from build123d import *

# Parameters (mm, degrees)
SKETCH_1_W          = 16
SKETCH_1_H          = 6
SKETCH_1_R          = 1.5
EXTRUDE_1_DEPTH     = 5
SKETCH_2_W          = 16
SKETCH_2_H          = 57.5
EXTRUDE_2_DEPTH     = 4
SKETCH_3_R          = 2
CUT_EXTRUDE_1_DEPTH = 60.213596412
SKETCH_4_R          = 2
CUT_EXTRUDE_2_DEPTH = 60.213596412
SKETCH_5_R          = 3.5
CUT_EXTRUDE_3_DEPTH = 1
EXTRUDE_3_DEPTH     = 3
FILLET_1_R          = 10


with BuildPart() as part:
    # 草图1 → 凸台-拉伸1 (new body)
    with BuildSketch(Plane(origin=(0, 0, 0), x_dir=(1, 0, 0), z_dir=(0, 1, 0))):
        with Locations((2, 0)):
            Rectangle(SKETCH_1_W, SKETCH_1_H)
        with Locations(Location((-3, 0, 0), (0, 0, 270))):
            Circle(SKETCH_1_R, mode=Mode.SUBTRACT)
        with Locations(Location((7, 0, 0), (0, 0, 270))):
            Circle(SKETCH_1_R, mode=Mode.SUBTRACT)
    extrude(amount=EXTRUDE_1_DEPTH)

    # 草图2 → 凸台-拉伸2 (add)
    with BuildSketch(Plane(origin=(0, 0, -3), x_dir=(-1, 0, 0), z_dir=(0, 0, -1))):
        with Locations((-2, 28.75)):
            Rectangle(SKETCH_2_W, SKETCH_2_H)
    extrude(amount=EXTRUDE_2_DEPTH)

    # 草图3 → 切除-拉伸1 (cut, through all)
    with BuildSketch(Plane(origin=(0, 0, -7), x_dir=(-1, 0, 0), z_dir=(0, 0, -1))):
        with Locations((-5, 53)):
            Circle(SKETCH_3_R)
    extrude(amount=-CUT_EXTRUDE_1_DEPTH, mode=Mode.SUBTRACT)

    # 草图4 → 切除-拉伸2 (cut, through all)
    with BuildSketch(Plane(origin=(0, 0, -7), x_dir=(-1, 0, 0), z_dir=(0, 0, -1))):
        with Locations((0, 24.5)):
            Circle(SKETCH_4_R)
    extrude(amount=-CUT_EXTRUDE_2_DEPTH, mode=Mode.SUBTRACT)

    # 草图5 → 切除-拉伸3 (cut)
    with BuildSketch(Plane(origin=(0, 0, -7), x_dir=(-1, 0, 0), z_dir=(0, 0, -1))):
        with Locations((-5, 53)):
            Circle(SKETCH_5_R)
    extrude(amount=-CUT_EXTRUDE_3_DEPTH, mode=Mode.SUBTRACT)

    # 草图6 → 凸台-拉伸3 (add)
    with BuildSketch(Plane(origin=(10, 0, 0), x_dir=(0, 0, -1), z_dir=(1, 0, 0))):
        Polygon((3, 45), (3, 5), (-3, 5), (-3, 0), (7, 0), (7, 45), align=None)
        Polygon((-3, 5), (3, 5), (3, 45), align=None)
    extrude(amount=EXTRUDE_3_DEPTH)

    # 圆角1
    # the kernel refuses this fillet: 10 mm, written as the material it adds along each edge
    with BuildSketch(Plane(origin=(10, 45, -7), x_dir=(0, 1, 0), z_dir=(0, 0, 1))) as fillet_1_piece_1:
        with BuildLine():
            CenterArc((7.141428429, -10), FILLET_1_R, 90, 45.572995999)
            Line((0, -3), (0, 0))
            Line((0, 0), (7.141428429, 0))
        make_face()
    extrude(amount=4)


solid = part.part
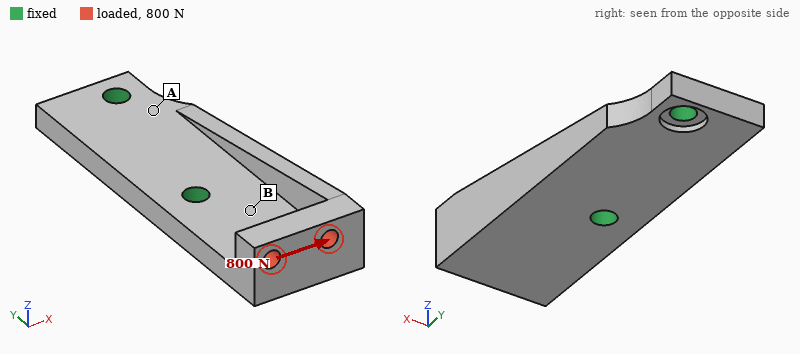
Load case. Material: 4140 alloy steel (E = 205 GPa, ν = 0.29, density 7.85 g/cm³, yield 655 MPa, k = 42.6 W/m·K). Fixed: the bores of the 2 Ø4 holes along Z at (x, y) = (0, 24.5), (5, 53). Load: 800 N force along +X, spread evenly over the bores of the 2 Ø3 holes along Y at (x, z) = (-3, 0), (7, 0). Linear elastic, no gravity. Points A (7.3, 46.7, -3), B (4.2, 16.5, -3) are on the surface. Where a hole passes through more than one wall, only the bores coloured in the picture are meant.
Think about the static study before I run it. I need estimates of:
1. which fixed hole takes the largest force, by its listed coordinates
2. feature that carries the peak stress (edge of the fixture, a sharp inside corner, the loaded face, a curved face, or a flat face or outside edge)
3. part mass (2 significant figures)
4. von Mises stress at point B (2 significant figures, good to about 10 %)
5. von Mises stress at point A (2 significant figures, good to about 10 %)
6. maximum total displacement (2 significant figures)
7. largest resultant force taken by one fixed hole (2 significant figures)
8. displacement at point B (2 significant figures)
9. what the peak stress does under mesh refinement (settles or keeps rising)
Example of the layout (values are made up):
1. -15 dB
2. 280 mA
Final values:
1. (0, 24.5)
2. edge of the fixture
3. 39 g
4. 81 MPa
5. 19 MPa
6. 48 µm
7. 1.3 kN
8. 7.6 µm
9. keeps rising
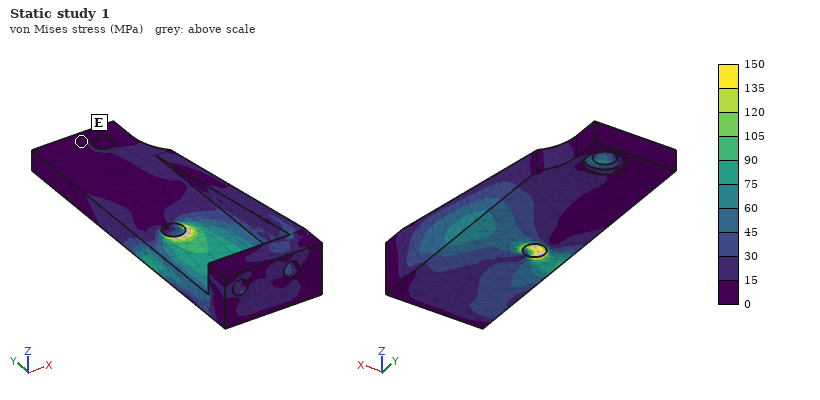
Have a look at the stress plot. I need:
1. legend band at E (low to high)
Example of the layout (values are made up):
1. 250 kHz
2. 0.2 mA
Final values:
1. 0 to 15 MPa
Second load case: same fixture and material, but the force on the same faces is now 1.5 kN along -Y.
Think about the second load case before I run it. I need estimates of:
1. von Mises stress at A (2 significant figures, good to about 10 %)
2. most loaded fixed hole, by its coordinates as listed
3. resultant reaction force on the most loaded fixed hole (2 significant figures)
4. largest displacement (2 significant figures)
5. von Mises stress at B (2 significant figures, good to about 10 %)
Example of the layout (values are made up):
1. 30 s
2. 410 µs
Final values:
1. 16 MPa
2. (0, 24.5)
3. 1.3 kN
4. 72 µm
5. 76 MPa
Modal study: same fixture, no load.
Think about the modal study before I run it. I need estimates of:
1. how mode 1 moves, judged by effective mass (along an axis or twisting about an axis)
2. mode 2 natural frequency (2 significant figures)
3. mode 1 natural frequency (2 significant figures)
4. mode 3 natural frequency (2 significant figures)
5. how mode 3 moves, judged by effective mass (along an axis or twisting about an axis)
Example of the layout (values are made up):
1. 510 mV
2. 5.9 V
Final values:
1. along Z
2. 8600 Hz
3. 4500 Hz
4. 12 kHz
5. along X
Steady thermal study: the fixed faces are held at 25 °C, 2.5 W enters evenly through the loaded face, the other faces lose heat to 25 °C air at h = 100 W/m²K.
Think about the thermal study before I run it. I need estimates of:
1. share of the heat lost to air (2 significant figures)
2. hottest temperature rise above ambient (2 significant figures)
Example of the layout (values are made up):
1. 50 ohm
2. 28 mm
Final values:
1. 47 %
2. 14 K
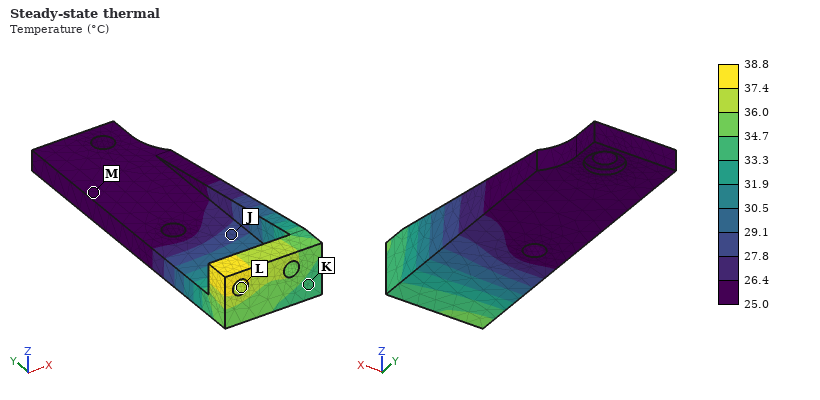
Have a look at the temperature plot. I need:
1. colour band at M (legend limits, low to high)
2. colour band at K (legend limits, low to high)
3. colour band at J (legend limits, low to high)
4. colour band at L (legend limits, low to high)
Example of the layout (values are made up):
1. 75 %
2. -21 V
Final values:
1. 25.0 to 26.4 °C
2. 33.3 to 34.7 °C
3. 27.8 to 29.1 °C
4. 36.0 to 37.4 °C
